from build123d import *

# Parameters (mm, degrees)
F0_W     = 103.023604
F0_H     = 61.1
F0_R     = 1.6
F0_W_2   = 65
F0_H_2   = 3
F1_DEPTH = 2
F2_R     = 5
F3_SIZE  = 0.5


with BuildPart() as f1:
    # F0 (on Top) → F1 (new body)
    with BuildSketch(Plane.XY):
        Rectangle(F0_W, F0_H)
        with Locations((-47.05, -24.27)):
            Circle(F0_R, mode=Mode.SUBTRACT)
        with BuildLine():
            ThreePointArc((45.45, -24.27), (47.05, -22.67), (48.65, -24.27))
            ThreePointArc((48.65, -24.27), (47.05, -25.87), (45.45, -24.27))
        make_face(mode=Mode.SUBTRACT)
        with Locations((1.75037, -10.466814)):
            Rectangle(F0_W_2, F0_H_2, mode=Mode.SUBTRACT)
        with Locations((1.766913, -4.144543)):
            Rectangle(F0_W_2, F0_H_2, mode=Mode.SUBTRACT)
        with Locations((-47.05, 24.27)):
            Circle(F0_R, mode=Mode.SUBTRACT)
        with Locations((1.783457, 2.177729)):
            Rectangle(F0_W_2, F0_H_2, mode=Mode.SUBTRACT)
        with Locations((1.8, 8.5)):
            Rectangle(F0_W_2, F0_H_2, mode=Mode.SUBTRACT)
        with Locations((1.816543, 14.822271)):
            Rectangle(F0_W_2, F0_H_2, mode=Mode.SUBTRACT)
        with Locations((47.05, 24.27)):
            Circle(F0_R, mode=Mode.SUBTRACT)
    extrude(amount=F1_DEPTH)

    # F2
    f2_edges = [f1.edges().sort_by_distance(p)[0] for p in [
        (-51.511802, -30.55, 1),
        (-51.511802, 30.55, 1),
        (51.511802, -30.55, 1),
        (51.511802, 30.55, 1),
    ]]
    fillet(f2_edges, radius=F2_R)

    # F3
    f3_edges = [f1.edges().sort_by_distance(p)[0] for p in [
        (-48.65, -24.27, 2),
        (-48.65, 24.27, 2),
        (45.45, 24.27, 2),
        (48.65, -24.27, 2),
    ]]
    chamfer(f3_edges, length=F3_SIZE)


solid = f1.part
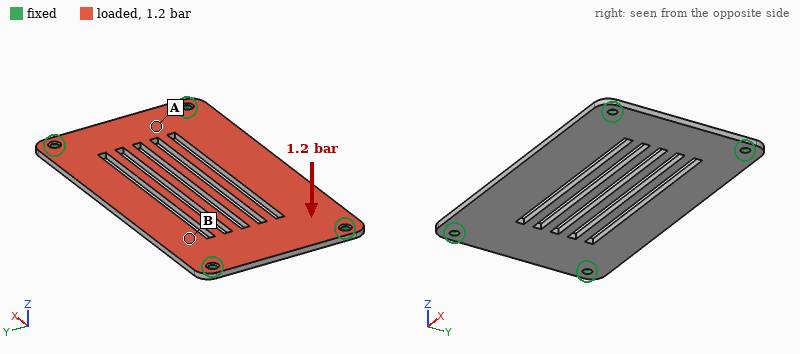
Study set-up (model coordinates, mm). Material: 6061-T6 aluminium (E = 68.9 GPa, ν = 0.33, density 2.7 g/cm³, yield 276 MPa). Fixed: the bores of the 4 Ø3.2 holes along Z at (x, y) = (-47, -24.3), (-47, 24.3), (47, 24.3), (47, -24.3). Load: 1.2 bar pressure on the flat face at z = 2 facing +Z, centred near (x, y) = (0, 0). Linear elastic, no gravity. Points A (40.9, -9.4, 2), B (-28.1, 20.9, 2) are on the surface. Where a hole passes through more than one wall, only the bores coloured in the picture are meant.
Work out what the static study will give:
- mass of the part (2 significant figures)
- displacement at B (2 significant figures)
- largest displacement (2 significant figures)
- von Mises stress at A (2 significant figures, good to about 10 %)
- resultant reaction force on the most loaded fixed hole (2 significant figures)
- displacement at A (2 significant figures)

28 g
0.29 mm
0.77 mm
46 MPa
170 N
0.14 mm
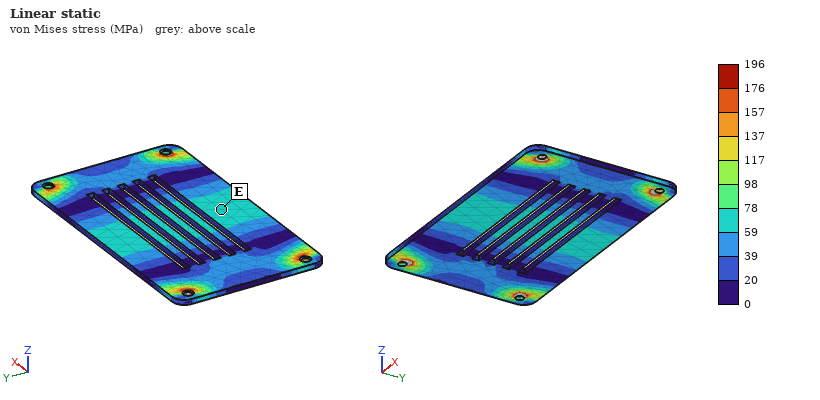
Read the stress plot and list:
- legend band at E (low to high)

59 to 78 MPa
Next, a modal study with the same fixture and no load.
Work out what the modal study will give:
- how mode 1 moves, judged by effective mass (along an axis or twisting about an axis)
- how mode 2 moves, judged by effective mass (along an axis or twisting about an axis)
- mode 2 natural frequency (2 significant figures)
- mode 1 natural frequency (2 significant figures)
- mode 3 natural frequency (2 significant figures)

along Z
twisting about X
1300 Hz
1100 Hz
1600 Hz
